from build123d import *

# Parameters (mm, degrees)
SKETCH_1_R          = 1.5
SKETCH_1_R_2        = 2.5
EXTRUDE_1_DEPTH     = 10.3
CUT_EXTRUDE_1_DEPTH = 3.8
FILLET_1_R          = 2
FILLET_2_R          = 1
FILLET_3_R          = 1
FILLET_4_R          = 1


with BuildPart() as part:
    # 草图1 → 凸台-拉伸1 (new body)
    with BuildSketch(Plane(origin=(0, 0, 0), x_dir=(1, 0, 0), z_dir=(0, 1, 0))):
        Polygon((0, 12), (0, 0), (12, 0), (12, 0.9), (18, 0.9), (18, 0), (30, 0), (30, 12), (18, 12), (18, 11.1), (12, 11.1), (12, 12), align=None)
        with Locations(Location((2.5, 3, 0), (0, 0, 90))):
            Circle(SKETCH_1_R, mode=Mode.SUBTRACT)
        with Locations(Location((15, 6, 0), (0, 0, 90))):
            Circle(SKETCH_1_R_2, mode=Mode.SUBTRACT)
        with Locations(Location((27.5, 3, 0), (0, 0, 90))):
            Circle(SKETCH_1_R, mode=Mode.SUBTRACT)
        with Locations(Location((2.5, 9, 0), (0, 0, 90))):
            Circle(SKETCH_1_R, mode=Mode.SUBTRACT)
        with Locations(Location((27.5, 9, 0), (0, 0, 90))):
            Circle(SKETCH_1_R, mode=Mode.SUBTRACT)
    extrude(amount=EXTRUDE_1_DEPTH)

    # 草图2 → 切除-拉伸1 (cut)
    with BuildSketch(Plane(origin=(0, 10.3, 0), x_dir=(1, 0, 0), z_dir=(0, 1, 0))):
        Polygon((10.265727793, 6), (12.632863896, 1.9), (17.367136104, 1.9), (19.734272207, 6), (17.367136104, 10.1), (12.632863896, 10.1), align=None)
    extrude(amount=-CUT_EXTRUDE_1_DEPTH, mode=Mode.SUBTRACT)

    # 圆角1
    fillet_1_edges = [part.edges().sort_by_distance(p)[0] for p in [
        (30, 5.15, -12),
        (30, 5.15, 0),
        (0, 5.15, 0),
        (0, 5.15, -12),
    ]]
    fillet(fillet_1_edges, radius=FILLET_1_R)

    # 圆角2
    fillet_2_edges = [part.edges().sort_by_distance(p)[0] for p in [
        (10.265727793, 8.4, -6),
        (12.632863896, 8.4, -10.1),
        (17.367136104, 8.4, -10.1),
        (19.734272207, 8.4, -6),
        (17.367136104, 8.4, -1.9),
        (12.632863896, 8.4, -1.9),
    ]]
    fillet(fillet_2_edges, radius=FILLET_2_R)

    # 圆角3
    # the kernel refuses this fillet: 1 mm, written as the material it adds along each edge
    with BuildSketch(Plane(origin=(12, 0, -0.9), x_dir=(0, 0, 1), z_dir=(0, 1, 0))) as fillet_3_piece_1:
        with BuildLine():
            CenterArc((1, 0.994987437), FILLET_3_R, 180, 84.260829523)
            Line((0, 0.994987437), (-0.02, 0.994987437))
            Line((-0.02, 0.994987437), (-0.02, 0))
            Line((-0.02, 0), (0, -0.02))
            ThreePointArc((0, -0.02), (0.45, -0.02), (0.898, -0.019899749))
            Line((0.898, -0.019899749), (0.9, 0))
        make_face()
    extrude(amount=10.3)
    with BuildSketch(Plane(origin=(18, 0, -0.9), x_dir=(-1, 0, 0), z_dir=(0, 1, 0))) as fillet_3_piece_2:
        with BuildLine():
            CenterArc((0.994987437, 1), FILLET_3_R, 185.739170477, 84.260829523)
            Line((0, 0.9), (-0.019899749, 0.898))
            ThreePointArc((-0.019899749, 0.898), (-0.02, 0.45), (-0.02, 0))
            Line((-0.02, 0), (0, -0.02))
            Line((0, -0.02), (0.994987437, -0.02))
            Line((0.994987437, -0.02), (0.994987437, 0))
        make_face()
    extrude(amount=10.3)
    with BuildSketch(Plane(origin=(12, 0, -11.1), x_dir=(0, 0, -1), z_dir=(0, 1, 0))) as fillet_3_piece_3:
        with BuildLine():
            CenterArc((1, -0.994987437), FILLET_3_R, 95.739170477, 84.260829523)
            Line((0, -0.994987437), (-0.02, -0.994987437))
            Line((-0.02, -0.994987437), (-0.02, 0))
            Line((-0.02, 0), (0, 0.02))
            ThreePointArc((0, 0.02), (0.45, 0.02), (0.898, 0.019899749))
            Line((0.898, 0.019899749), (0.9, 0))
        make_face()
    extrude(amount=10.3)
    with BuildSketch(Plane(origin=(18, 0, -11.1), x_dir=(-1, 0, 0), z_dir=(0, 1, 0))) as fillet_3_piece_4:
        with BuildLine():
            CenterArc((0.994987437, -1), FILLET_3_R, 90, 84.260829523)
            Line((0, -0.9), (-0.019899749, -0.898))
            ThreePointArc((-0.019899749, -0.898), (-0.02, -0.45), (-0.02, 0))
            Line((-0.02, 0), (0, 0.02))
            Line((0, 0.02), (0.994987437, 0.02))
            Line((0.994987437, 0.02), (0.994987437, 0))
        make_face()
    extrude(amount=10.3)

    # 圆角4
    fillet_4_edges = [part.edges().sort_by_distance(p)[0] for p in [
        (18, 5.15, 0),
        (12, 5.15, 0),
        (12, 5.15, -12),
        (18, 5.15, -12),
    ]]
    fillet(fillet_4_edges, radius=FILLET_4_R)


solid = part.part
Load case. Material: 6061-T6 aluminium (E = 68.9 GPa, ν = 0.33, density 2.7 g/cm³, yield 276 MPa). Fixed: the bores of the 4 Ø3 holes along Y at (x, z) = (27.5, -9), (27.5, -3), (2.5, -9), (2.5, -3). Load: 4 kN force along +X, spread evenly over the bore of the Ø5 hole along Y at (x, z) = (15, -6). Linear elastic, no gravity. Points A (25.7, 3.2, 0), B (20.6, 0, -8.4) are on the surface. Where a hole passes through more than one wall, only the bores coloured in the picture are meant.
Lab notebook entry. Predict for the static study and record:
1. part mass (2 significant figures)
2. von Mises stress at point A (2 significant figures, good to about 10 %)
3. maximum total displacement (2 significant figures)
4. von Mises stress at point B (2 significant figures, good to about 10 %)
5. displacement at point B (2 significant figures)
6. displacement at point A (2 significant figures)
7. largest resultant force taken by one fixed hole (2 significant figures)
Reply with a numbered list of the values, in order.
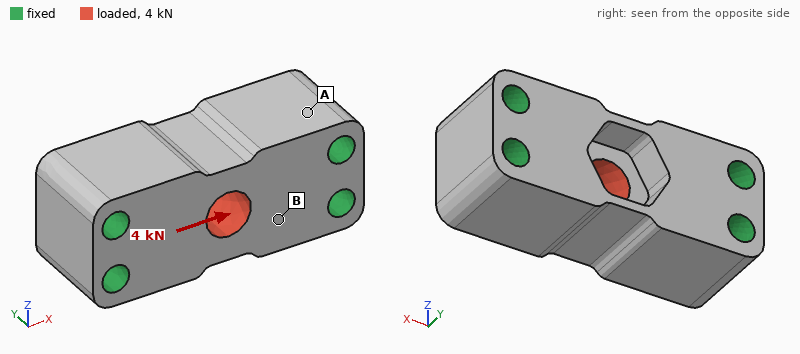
1. 7.9 g
2. 12 MPa
3. 4.4 µm
4. 31 MPa
5. 2.3 µm
6. 0.75 µm
7. 1.0 kN
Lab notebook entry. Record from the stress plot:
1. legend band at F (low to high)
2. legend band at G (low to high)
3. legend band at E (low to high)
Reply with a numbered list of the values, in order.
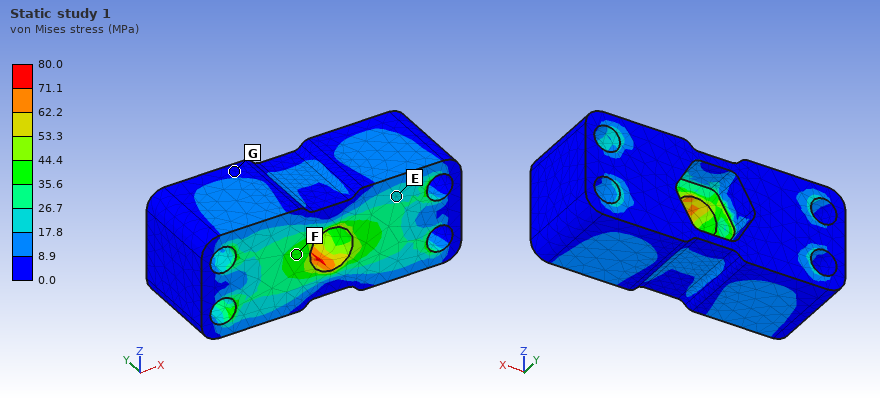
1. 35.6 to 44.4 MPa
2. 0.0 to 8.9 MPa
3. 17.8 to 26.7 MPa
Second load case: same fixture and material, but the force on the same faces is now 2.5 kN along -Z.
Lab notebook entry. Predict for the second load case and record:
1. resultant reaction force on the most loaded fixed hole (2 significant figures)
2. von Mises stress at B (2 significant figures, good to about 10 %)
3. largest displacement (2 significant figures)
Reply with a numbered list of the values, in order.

1. 1.2 kN
2. 35 MPa
3. 11 µm
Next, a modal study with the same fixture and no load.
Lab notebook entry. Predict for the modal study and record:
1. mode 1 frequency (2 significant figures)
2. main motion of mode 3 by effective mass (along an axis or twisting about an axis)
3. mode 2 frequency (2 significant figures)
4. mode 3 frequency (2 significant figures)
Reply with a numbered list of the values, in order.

1. 59 kHz
2. twisting about X
3. 60 kHz
4. 72 kHz
